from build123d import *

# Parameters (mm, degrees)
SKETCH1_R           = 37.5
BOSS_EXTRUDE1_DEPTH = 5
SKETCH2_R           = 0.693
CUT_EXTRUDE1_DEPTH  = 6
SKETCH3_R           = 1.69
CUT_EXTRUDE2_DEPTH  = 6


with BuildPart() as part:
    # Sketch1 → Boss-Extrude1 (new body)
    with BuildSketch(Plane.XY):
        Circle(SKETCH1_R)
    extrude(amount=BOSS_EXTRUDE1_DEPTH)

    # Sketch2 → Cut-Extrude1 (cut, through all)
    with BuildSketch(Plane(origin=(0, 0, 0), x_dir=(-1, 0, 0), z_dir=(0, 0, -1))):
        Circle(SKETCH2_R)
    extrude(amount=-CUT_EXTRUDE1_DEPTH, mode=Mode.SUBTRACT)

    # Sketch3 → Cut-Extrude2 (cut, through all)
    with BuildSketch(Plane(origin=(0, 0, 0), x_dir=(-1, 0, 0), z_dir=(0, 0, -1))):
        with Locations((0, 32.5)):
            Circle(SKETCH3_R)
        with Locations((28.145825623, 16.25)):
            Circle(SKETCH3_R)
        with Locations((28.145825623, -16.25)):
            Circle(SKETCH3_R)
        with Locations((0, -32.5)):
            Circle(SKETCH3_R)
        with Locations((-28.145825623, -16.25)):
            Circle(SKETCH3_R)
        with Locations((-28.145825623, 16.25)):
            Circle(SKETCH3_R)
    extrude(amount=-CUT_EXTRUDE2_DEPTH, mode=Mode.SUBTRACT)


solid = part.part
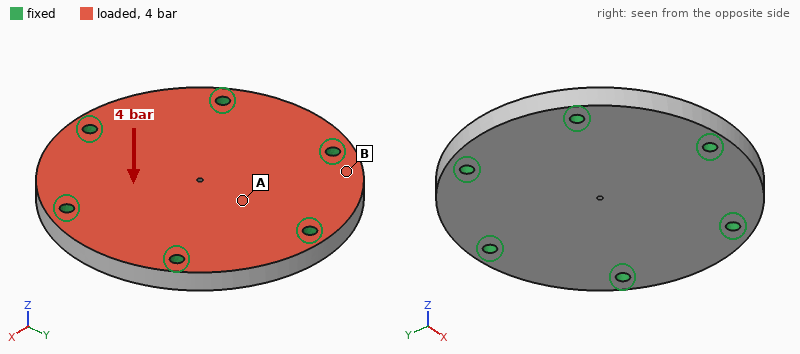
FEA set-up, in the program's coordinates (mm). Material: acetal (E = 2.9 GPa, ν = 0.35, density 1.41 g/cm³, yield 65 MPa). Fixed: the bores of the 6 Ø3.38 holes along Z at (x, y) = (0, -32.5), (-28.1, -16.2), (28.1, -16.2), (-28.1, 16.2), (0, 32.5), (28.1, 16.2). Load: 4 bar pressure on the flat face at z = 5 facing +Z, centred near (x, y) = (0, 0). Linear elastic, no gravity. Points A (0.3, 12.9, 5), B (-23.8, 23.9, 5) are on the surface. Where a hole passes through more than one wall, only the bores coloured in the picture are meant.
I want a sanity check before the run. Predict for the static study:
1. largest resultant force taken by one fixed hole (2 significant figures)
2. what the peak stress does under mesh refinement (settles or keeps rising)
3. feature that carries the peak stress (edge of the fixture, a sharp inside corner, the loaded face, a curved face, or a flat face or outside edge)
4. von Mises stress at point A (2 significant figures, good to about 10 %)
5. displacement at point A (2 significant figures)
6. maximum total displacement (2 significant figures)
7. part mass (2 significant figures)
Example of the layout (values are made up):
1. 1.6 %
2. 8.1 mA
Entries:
1. 290 N
2. keeps rising
3. edge of the fixture
4. 7.1 MPa
5. 0.25 mm
6. 0.32 mm
7. 31 g
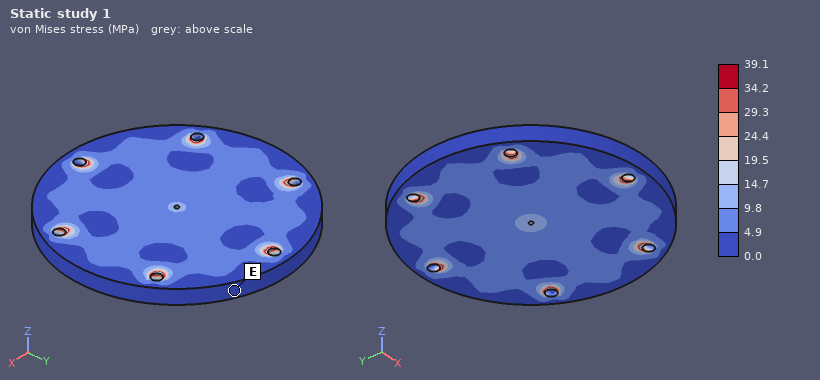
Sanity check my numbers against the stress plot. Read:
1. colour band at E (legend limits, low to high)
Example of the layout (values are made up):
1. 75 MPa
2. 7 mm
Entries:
1. 0.0 to 4.9 MPa
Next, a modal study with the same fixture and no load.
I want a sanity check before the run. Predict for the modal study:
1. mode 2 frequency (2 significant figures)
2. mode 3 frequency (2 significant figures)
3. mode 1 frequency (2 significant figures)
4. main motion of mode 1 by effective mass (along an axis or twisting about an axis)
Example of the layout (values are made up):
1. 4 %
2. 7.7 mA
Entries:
1. 5000 Hz
2. 5000 Hz
3. 2600 Hz
4. along Z
